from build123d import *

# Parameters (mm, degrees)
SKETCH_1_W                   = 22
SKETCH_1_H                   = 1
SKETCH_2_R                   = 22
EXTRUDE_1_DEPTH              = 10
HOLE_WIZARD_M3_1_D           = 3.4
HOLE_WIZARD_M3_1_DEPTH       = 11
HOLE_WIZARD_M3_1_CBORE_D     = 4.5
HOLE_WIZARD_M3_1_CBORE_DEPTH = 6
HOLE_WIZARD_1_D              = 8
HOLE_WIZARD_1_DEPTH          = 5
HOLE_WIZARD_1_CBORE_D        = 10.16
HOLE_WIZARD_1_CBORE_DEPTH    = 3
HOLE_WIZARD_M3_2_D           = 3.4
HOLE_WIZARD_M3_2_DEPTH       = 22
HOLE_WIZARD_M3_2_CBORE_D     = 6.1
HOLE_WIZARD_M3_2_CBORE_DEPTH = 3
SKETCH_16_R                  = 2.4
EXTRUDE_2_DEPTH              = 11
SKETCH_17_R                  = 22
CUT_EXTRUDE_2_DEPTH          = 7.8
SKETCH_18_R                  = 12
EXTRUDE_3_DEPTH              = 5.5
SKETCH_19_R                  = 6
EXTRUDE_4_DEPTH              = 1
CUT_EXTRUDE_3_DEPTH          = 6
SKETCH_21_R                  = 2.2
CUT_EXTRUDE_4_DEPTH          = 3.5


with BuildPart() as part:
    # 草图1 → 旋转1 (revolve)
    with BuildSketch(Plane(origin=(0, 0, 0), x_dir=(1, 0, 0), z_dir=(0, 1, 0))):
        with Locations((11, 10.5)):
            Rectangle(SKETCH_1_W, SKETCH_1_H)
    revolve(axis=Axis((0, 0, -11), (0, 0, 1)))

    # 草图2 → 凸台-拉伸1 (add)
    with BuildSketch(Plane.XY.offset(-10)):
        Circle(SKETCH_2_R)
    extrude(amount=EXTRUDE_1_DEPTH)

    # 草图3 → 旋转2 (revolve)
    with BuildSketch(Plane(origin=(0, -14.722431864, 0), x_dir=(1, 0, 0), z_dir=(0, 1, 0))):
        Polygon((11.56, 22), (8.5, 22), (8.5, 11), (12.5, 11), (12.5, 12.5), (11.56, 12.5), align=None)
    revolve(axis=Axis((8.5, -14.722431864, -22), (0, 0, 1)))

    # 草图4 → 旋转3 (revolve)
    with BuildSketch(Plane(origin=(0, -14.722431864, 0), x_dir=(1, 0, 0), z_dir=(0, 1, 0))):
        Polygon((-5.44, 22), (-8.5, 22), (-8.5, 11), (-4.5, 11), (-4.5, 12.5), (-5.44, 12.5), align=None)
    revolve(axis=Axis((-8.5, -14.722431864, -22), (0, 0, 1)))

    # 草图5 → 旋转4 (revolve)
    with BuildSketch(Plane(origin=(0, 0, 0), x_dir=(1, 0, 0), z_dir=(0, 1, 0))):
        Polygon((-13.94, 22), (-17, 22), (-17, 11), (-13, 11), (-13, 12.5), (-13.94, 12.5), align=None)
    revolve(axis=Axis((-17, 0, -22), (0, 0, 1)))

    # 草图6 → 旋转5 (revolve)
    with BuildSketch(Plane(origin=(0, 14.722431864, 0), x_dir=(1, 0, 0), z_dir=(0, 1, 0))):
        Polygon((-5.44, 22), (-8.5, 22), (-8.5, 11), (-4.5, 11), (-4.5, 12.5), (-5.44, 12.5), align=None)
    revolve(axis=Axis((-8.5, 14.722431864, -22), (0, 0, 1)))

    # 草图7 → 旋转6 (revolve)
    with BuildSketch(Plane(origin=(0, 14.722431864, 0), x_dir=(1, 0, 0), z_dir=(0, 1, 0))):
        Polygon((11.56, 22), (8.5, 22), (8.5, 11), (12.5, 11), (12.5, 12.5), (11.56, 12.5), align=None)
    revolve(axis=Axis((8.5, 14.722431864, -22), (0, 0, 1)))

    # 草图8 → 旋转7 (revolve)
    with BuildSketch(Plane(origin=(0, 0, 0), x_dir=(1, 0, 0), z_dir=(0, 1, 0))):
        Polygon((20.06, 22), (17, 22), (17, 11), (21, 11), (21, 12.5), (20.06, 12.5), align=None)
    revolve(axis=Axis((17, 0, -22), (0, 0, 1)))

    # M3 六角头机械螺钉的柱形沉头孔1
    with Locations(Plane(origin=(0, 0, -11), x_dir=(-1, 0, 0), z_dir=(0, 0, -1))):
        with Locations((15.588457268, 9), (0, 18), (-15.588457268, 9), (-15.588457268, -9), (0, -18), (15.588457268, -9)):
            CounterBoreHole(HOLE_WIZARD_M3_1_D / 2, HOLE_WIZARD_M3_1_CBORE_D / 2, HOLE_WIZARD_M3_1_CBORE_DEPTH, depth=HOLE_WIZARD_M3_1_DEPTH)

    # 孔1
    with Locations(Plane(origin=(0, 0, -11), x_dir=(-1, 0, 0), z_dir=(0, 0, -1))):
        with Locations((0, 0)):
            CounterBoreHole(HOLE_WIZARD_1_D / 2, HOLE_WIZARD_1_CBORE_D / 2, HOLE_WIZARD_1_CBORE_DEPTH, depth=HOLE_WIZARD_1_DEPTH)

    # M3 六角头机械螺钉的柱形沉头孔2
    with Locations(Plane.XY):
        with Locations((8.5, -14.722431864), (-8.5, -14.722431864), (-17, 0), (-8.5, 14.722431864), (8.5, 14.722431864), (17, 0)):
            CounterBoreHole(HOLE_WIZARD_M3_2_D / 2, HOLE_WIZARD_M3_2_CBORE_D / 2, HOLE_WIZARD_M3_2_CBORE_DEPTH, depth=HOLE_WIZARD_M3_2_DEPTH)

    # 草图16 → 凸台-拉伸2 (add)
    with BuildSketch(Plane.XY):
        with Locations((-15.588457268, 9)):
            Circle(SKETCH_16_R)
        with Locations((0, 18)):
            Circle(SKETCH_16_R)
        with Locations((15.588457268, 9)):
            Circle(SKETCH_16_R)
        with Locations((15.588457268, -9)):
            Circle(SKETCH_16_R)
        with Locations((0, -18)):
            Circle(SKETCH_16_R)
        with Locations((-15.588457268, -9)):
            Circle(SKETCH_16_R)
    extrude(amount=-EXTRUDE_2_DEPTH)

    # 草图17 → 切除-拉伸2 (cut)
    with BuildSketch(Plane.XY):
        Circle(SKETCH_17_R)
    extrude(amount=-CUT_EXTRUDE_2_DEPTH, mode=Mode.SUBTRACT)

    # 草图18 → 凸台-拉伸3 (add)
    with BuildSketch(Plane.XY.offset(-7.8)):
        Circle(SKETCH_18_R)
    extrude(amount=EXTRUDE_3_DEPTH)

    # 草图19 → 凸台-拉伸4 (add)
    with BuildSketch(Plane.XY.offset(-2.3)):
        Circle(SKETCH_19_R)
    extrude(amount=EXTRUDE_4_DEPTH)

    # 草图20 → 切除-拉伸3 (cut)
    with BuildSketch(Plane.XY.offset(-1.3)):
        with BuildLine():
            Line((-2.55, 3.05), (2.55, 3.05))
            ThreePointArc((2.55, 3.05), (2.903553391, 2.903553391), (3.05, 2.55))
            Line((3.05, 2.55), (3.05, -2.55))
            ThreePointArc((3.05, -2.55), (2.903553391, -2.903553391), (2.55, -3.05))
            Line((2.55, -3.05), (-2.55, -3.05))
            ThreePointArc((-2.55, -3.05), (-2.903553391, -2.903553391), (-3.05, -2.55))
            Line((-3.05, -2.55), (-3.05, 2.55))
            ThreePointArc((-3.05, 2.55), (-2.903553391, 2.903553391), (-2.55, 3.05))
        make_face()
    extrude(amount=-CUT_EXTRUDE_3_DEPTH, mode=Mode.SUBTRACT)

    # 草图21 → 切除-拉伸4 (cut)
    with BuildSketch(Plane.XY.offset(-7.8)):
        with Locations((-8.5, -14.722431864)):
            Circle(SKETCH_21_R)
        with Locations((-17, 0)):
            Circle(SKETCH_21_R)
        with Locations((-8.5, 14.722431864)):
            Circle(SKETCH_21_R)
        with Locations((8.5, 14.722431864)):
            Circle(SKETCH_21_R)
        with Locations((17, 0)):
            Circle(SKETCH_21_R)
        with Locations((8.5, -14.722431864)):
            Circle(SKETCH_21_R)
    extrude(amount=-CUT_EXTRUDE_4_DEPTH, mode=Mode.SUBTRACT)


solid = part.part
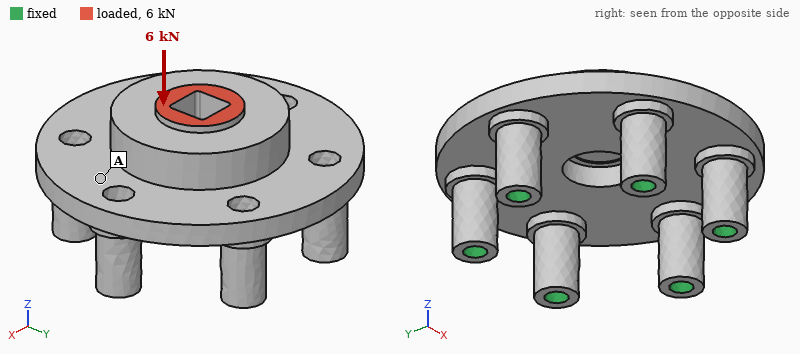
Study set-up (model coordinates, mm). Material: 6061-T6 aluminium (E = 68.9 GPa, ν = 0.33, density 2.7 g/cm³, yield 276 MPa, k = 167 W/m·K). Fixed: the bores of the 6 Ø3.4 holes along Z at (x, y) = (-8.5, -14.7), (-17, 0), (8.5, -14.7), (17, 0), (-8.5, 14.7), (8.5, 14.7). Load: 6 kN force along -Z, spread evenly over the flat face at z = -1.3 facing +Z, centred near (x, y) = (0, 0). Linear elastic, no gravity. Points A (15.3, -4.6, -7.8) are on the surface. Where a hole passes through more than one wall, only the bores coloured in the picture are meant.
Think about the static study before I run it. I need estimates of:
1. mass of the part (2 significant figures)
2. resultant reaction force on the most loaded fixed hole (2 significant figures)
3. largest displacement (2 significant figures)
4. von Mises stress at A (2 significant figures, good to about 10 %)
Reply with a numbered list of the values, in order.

1. 22 g
2. 1.4 kN
3. 28 µm
4. 20 MPa
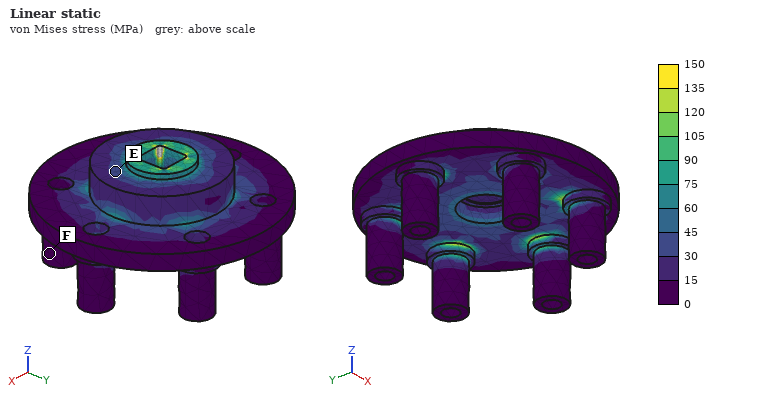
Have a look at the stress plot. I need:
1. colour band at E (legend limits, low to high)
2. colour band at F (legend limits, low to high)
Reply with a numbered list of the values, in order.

1. 30 to 45 MPa
2. 0 to 15 MPa
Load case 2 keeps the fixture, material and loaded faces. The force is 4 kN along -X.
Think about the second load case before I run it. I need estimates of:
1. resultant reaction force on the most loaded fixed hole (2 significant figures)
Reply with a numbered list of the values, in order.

1. 1.3 kN
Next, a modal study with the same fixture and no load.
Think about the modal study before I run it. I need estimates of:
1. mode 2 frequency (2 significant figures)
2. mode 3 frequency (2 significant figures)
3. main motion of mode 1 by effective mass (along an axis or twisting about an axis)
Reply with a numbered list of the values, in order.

1. 33 kHz
2. 33 kHz
3. along Z
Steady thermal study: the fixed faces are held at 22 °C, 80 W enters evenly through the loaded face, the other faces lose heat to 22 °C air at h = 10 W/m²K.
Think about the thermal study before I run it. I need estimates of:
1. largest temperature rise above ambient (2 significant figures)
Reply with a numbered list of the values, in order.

1. 43 K
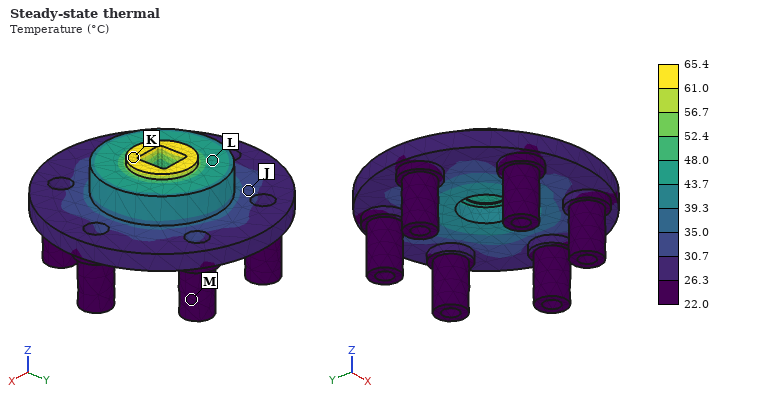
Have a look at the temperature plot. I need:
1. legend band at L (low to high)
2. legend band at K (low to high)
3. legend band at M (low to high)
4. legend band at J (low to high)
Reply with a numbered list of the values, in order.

1. 43.7 to 48.0 °C
2. 61.0 to 65.4 °C
3. 22.0 to 26.3 °C
4. 30.7 to 35.0 °C
